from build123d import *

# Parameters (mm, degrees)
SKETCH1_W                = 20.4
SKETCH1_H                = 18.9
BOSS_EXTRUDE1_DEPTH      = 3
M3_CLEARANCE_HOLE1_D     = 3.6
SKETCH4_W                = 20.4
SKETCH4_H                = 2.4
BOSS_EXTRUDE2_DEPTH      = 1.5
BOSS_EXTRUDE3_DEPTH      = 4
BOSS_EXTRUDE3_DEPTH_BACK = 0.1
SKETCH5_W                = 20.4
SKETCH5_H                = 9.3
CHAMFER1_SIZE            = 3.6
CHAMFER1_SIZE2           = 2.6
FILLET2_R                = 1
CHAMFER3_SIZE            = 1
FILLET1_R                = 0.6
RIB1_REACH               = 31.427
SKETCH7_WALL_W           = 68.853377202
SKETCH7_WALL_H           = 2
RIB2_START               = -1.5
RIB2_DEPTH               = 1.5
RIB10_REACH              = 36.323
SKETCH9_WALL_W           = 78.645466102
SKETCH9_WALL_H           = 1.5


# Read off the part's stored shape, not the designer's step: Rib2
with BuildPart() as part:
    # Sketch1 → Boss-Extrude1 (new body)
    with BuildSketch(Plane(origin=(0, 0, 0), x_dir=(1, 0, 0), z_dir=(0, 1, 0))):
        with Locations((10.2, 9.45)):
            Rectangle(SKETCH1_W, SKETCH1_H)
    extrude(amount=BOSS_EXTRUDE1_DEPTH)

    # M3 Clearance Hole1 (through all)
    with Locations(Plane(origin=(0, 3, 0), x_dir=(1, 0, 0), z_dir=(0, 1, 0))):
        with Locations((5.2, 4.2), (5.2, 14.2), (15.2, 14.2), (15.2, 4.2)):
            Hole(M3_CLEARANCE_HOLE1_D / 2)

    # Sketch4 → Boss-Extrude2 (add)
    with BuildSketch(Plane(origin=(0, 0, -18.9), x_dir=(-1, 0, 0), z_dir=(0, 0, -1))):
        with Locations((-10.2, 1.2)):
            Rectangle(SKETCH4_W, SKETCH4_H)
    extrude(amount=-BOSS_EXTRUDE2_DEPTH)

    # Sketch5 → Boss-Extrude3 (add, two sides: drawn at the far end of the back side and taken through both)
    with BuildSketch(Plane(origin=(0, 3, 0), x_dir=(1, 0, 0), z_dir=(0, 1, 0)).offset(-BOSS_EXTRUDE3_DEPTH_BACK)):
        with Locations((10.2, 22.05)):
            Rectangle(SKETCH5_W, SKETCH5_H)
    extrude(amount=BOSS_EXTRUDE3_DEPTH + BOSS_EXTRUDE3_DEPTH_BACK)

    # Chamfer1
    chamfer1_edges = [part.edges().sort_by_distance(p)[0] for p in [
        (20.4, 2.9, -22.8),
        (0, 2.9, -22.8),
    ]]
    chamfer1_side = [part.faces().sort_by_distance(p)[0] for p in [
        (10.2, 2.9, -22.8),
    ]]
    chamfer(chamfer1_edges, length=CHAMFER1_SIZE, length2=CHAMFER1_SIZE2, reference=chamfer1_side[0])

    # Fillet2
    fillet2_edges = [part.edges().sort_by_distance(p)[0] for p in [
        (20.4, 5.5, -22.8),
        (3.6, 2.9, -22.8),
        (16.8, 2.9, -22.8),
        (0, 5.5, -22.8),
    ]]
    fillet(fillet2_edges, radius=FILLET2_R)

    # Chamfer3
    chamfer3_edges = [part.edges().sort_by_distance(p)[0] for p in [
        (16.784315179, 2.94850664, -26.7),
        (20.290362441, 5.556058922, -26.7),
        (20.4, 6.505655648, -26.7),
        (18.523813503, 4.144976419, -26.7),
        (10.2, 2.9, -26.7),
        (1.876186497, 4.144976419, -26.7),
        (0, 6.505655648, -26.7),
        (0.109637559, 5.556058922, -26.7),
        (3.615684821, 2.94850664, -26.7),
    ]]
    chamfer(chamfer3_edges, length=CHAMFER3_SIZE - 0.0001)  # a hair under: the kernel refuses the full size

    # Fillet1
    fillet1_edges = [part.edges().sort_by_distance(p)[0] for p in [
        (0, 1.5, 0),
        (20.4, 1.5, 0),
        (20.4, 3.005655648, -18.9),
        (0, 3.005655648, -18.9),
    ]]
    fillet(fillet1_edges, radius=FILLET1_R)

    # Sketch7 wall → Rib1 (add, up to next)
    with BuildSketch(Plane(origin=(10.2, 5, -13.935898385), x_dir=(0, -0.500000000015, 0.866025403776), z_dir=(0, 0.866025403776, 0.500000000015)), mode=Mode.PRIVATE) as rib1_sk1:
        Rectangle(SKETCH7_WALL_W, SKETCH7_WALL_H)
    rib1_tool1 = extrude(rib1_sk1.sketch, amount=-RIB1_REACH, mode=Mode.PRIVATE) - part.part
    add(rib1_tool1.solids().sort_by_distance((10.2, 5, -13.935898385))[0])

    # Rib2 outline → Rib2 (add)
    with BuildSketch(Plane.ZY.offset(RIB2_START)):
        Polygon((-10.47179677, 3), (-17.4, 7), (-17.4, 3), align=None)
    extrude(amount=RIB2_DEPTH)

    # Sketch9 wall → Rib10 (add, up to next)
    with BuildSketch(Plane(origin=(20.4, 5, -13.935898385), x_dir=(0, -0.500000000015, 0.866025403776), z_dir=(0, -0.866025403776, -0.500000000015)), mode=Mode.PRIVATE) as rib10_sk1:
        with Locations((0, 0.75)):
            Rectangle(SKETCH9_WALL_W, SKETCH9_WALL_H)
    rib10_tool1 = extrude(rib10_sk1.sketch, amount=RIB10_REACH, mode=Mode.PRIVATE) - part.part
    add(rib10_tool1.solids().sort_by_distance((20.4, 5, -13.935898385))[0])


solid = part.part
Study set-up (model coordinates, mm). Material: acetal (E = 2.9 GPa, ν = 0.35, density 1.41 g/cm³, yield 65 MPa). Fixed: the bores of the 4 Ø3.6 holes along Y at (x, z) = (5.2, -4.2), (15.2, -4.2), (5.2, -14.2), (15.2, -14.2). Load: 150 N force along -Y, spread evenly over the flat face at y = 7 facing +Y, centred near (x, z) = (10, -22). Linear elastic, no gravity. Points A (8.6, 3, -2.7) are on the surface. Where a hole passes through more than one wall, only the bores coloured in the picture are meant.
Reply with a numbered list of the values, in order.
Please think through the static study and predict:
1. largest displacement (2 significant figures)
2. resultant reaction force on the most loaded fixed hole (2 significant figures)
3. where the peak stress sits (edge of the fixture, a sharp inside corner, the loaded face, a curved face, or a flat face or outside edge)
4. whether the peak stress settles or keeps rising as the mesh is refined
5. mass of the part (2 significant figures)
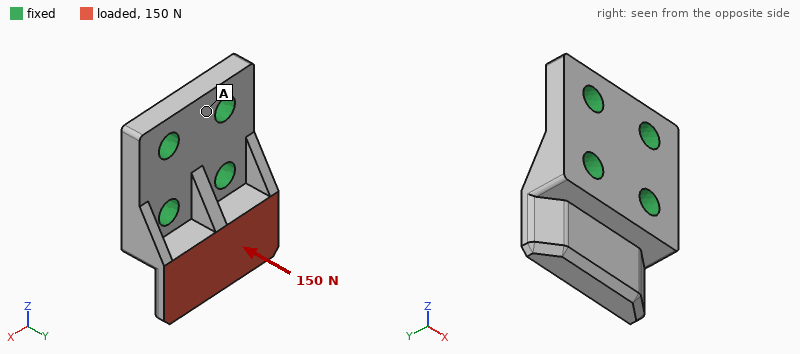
1. 0.27 mm
2. 92 N
3. edge of the fixture
4. keeps rising
5. 2.5 g
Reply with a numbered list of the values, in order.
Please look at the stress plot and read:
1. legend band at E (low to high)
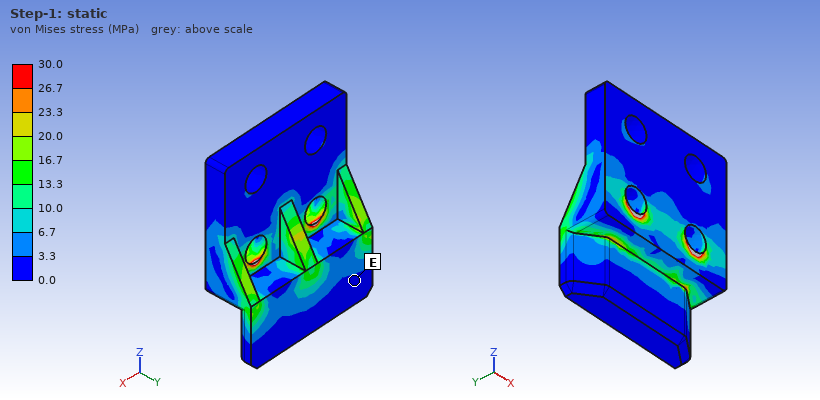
1. 0.0 to 3.3 MPa
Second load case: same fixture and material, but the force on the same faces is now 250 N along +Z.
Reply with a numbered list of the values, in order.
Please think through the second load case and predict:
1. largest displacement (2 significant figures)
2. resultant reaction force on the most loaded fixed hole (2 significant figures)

1. 0.36 mm
2. 90 N
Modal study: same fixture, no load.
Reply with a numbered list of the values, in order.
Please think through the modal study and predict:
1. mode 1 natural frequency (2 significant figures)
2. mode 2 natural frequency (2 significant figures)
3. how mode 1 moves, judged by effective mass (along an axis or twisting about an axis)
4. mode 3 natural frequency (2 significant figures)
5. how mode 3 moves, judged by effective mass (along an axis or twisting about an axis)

1. 4600 Hz
2. 8100 Hz
3. along Y
4. 11 kHz
5. along X
